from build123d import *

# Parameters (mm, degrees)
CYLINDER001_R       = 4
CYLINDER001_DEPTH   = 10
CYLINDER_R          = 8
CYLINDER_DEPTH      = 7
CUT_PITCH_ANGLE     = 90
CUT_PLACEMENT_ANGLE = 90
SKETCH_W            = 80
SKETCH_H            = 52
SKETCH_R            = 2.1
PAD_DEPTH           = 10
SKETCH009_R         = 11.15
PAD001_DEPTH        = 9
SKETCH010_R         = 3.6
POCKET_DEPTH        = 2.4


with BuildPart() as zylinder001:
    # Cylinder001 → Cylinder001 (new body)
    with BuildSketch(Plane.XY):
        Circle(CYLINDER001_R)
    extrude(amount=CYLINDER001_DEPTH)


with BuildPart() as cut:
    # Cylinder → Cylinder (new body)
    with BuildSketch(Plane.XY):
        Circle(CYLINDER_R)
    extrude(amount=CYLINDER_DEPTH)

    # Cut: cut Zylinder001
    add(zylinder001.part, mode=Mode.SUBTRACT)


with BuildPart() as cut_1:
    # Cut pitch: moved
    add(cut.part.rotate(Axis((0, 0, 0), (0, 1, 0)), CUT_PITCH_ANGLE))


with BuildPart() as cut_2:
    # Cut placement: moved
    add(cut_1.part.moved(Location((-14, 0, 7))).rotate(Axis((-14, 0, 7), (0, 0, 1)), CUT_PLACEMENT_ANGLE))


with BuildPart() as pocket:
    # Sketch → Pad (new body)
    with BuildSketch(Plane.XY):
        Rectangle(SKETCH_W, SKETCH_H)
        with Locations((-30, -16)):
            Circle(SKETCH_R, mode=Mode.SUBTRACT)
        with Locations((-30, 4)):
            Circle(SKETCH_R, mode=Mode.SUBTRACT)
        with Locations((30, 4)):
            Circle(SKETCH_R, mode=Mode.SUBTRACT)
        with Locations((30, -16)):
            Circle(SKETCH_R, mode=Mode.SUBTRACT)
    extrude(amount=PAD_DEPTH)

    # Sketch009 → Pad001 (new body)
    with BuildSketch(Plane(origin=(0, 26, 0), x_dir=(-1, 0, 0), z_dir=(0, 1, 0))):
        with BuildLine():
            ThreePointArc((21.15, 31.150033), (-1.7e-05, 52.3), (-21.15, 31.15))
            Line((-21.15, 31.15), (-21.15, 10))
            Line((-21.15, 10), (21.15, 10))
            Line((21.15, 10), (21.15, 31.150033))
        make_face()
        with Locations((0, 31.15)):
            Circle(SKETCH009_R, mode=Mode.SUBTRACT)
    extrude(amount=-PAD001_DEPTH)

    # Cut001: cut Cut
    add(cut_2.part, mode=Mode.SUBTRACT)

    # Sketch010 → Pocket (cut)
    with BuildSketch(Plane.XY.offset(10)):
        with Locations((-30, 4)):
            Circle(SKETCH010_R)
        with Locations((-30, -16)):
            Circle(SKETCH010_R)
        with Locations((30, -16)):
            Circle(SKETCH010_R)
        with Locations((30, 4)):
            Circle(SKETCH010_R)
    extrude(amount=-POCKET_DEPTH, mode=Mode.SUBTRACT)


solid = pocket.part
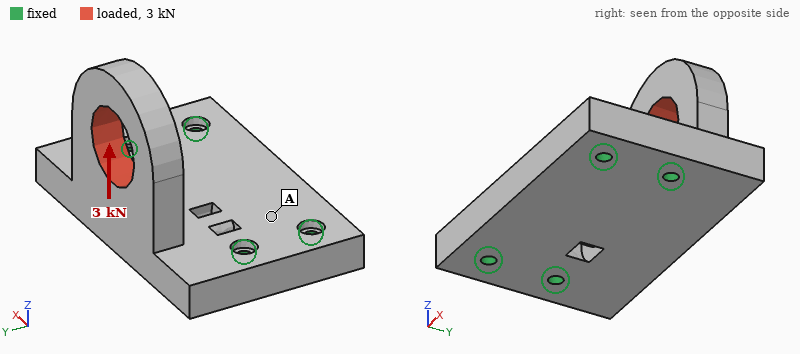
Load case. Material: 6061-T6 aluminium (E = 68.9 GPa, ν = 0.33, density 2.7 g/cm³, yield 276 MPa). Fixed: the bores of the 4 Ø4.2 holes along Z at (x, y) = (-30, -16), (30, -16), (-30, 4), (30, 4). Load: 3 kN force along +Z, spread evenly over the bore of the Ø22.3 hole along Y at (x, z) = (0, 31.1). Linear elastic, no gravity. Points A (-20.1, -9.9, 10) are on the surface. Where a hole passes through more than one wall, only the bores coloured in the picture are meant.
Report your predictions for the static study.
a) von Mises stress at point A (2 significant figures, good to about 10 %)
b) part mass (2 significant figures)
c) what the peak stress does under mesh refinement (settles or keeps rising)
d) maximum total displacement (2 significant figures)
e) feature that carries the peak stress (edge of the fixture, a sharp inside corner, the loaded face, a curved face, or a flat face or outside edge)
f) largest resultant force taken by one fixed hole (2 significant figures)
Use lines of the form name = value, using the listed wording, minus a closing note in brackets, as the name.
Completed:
von Mises stress at point A = 17 MPa
part mass = 140 g
what the peak stress does under mesh refinement = keeps rising
maximum total displacement = 0.12 mm
feature that carries the peak stress = edge of the fixture
largest resultant force taken by one fixed hole = 2.3 kN
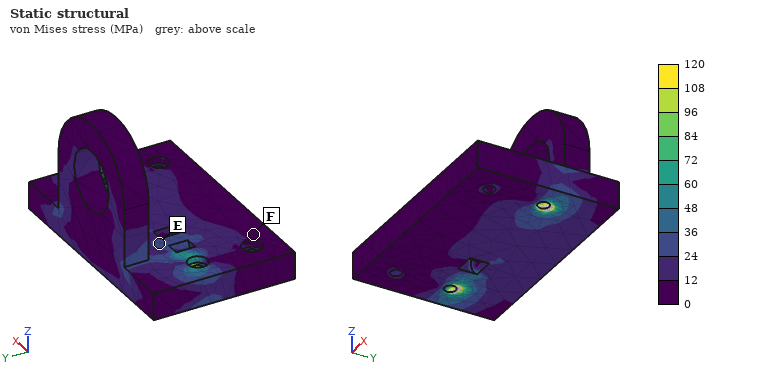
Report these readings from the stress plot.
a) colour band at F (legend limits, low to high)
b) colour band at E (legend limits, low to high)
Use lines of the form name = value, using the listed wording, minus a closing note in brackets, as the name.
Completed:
colour band at F = 0 to 12 MPa
colour band at E = 24 to 36 MPa
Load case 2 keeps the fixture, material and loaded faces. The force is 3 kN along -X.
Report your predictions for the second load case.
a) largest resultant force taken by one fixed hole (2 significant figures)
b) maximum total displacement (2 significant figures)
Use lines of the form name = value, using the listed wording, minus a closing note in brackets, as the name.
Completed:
largest resultant force taken by one fixed hole = 2.3 kN
maximum total displacement = 90 µm
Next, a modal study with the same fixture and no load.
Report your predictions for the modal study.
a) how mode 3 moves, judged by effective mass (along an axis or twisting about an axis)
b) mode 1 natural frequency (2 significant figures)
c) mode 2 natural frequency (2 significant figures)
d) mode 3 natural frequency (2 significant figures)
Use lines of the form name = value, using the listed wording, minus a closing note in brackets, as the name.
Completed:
how mode 3 moves, judged by effective mass = along Z
mode 1 natural frequency = 2900 Hz
mode 2 natural frequency = 6100 Hz
mode 3 natural frequency = 6600 Hz
